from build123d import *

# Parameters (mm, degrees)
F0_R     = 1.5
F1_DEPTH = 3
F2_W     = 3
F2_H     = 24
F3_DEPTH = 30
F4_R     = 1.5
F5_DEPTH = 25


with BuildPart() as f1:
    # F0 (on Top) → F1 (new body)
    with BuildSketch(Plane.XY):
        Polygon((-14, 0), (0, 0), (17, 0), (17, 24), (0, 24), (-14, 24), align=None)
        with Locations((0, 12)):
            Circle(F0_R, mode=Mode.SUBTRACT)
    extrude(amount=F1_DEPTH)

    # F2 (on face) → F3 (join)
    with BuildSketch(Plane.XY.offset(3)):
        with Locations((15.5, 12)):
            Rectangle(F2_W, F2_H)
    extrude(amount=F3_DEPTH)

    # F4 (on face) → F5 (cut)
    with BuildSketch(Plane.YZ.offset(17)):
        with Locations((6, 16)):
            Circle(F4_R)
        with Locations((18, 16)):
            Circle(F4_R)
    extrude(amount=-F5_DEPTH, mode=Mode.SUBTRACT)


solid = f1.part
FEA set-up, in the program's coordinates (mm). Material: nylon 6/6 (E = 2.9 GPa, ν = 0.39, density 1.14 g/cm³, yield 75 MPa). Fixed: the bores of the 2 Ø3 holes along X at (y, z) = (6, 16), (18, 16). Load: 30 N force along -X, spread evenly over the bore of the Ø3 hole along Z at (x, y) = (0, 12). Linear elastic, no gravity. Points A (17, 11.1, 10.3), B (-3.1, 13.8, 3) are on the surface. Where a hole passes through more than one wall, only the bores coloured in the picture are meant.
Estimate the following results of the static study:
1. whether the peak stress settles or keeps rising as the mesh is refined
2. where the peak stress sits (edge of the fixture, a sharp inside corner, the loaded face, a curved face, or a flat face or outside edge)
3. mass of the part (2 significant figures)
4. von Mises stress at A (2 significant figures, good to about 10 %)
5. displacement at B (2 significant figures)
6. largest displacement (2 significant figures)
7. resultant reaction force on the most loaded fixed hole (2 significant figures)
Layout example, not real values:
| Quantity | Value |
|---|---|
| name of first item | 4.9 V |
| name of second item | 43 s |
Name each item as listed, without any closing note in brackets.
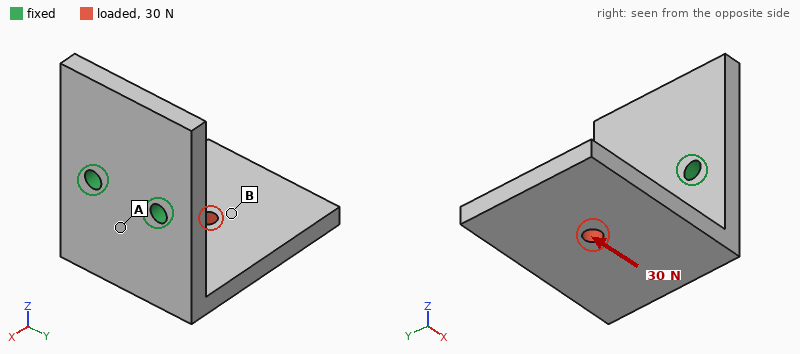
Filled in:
| Quantity | Value |
|---|---|
| whether the peak stress settles or keeps rising as the mesh is refined | keeps rising |
| where the peak stress sits | edge of the fixture |
| mass of the part | 4.9 g |
| von Mises stress at A | 6.2 MPa |
| displacement at B | 0.37 mm |
| largest displacement | 0.57 mm |
| resultant reaction force on the most loaded fixed hole | 15 N |
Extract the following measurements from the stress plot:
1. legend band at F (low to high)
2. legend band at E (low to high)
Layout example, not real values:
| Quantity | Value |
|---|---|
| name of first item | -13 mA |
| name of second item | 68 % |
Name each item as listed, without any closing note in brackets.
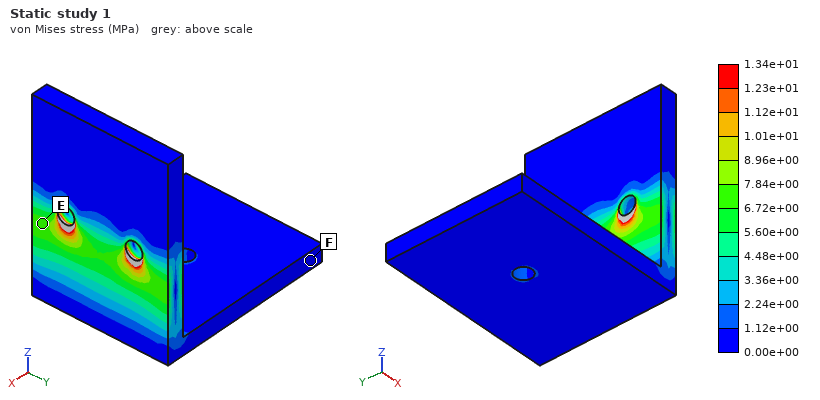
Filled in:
| Quantity | Value |
|---|---|
| legend band at F | 0.00e+00 to 1.12e+00 MPa |
| legend band at E | 6.72e+00 to 7.84e+00 MPa |
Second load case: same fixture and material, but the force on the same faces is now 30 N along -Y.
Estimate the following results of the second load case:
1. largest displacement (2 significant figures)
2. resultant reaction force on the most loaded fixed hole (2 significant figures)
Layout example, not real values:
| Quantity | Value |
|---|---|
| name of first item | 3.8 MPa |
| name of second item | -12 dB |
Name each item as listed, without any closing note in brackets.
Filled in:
| Quantity | Value |
|---|---|
| largest displacement | 0.50 mm |
| resultant reaction force on the most loaded fixed hole | 45 N |
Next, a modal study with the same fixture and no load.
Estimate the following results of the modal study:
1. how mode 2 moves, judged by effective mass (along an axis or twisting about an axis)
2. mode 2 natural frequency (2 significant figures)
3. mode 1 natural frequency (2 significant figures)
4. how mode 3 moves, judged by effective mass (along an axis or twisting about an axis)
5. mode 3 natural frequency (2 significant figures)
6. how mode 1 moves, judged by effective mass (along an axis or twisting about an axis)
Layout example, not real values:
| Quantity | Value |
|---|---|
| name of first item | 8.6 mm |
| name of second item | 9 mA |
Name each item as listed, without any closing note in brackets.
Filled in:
| Quantity | Value |
|---|---|
| how mode 2 moves, judged by effective mass | along Y |
| mode 2 natural frequency | 960 Hz |
| mode 1 natural frequency | 530 Hz |
| how mode 3 moves, judged by effective mass | along X |
| mode 3 natural frequency | 1800 Hz |
| how mode 1 moves, judged by effective mass | along Z |
